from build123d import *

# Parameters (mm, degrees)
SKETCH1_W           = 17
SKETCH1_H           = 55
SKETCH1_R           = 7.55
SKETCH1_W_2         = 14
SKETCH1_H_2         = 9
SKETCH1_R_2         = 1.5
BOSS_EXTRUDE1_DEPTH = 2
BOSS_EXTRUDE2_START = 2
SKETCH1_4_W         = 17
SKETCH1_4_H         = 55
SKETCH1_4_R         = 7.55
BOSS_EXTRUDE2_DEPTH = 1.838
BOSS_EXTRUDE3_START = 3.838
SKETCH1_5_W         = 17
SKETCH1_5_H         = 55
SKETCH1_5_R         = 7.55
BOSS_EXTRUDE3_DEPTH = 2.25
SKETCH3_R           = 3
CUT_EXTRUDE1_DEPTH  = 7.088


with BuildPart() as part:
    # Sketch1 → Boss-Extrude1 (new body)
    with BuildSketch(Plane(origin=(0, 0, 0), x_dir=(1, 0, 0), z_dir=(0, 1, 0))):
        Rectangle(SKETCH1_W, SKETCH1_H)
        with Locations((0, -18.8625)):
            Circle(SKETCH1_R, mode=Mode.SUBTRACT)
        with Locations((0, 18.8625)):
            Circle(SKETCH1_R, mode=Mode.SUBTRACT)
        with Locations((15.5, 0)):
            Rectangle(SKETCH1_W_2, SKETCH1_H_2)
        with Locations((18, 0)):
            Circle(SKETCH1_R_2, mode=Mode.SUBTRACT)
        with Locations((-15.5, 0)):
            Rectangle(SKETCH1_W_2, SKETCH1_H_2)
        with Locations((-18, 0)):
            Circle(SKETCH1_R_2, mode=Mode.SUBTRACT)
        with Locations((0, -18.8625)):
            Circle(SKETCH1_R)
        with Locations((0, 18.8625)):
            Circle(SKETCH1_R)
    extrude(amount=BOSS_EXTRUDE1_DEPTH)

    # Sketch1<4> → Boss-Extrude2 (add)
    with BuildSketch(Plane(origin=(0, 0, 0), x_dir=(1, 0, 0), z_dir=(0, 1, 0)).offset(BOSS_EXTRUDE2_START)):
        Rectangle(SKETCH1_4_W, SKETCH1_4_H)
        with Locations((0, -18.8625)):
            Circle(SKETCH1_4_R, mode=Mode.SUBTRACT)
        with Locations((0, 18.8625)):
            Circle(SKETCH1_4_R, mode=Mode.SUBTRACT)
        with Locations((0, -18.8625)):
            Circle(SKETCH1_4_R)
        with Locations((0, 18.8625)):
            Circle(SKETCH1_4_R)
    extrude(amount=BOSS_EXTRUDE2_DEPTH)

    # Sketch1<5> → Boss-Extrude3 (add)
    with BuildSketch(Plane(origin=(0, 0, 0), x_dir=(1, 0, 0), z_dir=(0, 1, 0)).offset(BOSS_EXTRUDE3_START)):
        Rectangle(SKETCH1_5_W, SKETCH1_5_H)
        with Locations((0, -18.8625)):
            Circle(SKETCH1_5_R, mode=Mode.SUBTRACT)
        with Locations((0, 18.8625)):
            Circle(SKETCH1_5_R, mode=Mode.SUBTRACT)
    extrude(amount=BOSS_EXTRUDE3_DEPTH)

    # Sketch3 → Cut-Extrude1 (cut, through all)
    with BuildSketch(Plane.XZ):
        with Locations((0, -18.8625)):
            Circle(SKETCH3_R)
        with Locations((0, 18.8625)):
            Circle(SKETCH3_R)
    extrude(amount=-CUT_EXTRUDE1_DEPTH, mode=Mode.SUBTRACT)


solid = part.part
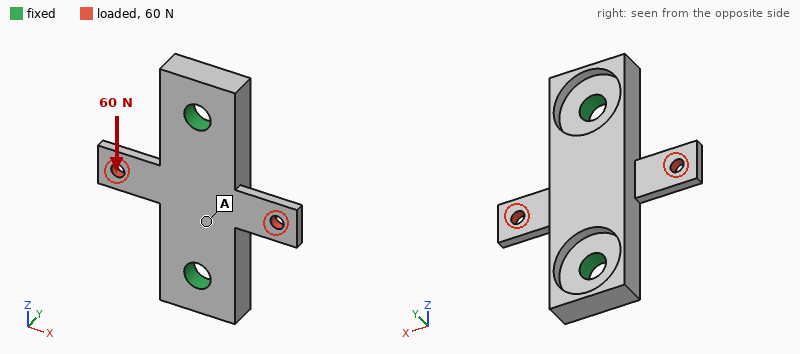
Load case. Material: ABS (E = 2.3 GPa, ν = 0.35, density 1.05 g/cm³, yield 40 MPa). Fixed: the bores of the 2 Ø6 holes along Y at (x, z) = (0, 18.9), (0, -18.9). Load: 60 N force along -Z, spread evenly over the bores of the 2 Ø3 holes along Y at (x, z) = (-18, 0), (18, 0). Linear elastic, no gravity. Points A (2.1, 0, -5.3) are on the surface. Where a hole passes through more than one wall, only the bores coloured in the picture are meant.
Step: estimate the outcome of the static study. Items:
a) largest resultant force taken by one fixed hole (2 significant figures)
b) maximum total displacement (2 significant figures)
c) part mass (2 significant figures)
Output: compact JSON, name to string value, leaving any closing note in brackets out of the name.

{"largest resultant force taken by one fixed hole": "30 N", "maximum total displacement": "0.13 mm", "part mass": "5.4 g"}
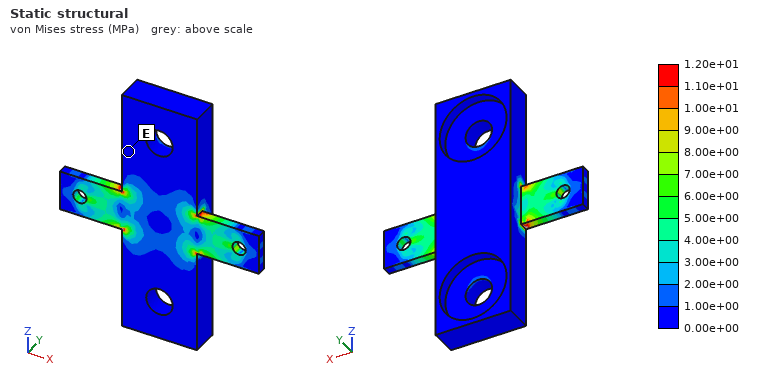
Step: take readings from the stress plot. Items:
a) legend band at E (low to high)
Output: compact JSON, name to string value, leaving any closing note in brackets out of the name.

{"legend band at E": "0.00e+00 to 1.00e+00 MPa"}
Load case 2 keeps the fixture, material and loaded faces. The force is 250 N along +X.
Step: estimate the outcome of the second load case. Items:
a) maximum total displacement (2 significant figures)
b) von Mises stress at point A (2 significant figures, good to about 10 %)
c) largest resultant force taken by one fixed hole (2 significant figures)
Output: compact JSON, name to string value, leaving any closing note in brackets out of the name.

{"maximum total displacement": "0.18 mm", "von Mises stress at point A": "4.3 MPa", "largest resultant force taken by one fixed hole": "130 N"}
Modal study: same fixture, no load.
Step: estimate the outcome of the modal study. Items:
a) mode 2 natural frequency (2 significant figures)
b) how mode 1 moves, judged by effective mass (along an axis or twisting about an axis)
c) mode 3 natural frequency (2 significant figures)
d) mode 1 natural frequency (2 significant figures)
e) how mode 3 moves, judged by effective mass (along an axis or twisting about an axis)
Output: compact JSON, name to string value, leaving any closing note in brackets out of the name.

{"mode 2 natural frequency": "2100 Hz", "how mode 1 moves, judged by effective mass": "twisting about Z", "mode 3 natural frequency": "4900 Hz", "mode 1 natural frequency": "2000 Hz", "how mode 3 moves, judged by effective mass": "along Y"}
